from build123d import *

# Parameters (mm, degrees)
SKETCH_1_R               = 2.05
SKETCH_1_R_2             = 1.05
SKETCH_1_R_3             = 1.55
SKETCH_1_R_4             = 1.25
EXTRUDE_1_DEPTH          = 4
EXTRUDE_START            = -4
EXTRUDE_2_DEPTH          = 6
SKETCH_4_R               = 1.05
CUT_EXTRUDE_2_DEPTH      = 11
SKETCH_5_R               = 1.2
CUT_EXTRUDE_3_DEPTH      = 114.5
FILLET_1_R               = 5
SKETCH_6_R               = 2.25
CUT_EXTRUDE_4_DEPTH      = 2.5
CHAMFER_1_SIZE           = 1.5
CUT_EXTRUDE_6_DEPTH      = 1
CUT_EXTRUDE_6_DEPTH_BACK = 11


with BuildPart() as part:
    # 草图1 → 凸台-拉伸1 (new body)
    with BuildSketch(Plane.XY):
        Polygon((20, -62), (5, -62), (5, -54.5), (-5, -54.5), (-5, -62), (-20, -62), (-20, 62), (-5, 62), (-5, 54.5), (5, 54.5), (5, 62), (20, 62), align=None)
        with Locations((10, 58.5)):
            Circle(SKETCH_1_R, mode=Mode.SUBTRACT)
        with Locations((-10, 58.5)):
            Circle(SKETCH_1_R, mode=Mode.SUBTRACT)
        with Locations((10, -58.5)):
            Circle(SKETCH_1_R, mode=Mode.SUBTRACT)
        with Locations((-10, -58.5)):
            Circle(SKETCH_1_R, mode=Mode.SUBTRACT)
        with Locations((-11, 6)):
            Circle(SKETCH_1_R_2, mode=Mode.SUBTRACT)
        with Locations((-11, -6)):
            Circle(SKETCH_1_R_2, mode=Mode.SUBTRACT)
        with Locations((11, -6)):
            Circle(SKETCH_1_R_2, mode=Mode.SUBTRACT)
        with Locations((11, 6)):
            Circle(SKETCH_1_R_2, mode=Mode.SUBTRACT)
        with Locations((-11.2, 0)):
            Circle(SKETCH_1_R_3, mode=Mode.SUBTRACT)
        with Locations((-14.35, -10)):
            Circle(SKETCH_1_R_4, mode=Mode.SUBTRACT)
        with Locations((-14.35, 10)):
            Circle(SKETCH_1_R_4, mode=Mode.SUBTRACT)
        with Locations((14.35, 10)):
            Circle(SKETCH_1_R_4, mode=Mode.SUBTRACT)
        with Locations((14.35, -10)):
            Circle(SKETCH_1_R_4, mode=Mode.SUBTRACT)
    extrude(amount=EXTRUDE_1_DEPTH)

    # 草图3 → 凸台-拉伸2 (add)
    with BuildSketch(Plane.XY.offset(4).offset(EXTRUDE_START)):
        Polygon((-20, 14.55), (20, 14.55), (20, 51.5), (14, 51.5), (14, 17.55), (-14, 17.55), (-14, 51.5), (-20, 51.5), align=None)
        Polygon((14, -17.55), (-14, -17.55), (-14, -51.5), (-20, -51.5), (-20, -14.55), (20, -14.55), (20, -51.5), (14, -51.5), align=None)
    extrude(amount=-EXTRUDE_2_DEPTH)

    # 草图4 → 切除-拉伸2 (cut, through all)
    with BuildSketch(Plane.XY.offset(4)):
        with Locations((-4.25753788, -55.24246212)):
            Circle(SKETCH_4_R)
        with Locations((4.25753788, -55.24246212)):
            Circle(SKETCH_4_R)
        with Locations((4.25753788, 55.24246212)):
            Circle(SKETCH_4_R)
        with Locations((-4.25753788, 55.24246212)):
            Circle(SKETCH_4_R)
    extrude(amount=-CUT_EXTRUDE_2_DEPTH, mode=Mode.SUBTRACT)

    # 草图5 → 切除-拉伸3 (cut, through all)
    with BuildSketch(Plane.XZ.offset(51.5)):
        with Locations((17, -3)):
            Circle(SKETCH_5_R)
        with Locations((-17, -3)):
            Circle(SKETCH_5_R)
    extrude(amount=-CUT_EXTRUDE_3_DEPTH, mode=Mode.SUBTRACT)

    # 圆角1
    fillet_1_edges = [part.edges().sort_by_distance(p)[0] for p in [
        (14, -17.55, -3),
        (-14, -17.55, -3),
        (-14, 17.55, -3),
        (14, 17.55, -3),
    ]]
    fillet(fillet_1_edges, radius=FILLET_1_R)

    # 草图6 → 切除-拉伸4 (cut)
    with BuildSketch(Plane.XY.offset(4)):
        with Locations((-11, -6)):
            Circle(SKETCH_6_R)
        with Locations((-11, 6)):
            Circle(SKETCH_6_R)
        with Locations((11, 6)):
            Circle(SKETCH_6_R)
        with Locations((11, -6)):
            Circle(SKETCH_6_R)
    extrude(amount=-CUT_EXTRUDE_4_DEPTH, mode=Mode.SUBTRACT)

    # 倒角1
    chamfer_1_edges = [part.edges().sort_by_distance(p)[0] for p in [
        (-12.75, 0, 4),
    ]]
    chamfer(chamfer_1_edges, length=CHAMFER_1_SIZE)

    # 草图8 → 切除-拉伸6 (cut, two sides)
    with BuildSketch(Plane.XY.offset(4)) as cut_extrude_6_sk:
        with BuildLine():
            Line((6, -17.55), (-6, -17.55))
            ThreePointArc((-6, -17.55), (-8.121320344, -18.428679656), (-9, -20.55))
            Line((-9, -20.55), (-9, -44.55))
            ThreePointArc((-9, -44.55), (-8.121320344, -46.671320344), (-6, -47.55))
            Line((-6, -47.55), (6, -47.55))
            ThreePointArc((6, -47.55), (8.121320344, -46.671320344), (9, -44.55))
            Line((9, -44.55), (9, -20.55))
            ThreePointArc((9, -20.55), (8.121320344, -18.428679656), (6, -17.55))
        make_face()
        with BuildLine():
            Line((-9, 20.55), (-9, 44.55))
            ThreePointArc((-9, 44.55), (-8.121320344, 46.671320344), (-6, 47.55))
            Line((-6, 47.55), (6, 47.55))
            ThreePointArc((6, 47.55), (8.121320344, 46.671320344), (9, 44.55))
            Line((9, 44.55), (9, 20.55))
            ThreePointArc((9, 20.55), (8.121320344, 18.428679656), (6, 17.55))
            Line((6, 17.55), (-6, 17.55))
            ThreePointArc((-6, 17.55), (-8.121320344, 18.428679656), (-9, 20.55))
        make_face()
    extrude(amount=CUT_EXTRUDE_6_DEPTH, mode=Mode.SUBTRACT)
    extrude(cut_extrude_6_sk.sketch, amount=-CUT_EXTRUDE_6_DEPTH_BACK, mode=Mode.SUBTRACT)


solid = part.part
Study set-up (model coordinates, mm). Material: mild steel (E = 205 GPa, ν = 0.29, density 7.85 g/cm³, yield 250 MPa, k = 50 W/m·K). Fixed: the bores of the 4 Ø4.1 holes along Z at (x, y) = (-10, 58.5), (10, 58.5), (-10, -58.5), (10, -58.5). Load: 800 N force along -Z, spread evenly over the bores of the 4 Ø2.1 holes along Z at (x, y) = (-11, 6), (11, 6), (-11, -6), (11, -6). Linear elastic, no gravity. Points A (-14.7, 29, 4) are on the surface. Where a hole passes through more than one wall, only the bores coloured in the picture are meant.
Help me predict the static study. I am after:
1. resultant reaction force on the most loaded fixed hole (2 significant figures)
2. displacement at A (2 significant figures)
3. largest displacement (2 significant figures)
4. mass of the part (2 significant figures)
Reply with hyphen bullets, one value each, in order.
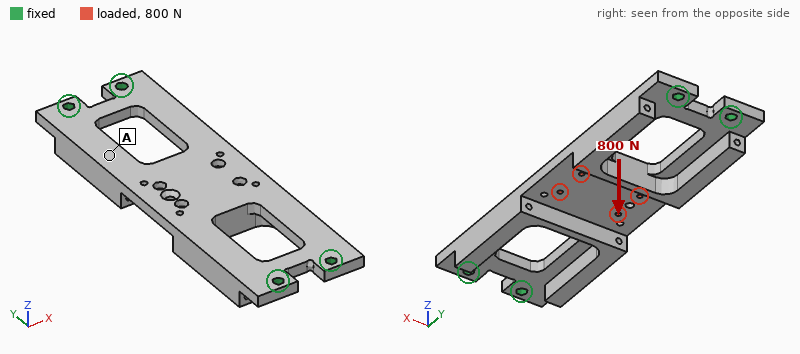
- 210 N
- 0.084 mm
- 0.16 mm
- 160 g
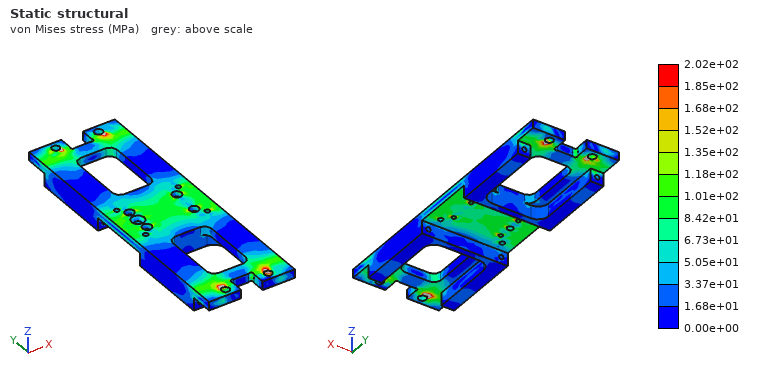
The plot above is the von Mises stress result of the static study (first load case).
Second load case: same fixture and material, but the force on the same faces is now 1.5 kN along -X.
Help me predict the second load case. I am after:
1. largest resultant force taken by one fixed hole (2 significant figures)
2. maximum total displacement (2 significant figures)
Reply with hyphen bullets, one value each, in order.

- 450 N
- 33 µm
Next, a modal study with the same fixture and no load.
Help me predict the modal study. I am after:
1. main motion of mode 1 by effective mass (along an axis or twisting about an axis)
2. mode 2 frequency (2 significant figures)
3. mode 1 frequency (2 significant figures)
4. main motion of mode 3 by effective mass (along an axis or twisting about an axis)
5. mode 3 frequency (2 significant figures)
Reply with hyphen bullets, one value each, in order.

- along Z
- 2800 Hz
- 1400 Hz
- along X
- 4000 Hz
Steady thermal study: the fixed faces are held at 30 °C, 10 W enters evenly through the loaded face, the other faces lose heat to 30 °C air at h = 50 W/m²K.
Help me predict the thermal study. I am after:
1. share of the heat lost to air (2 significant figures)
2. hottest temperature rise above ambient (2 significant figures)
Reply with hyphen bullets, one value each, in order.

- 64 %
- 27 K
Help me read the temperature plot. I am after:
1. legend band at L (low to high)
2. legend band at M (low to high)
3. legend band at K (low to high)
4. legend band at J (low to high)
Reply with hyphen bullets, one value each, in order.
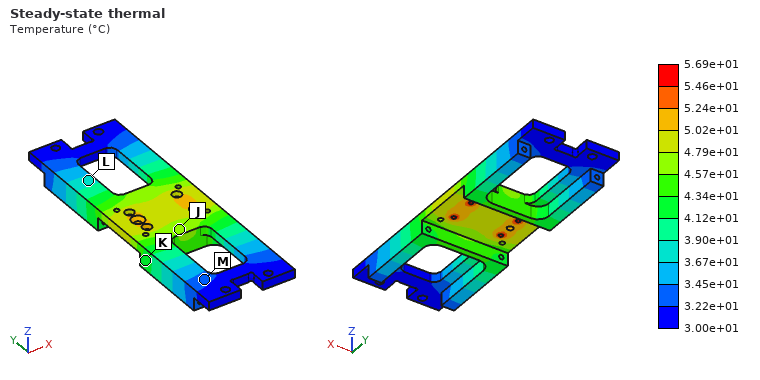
- 3.67e+01 to 3.90e+01 °C
- 3.22e+01 to 3.45e+01 °C
- 4.12e+01 to 4.34e+01 °C
- 4.57e+01 to 4.79e+01 °C
